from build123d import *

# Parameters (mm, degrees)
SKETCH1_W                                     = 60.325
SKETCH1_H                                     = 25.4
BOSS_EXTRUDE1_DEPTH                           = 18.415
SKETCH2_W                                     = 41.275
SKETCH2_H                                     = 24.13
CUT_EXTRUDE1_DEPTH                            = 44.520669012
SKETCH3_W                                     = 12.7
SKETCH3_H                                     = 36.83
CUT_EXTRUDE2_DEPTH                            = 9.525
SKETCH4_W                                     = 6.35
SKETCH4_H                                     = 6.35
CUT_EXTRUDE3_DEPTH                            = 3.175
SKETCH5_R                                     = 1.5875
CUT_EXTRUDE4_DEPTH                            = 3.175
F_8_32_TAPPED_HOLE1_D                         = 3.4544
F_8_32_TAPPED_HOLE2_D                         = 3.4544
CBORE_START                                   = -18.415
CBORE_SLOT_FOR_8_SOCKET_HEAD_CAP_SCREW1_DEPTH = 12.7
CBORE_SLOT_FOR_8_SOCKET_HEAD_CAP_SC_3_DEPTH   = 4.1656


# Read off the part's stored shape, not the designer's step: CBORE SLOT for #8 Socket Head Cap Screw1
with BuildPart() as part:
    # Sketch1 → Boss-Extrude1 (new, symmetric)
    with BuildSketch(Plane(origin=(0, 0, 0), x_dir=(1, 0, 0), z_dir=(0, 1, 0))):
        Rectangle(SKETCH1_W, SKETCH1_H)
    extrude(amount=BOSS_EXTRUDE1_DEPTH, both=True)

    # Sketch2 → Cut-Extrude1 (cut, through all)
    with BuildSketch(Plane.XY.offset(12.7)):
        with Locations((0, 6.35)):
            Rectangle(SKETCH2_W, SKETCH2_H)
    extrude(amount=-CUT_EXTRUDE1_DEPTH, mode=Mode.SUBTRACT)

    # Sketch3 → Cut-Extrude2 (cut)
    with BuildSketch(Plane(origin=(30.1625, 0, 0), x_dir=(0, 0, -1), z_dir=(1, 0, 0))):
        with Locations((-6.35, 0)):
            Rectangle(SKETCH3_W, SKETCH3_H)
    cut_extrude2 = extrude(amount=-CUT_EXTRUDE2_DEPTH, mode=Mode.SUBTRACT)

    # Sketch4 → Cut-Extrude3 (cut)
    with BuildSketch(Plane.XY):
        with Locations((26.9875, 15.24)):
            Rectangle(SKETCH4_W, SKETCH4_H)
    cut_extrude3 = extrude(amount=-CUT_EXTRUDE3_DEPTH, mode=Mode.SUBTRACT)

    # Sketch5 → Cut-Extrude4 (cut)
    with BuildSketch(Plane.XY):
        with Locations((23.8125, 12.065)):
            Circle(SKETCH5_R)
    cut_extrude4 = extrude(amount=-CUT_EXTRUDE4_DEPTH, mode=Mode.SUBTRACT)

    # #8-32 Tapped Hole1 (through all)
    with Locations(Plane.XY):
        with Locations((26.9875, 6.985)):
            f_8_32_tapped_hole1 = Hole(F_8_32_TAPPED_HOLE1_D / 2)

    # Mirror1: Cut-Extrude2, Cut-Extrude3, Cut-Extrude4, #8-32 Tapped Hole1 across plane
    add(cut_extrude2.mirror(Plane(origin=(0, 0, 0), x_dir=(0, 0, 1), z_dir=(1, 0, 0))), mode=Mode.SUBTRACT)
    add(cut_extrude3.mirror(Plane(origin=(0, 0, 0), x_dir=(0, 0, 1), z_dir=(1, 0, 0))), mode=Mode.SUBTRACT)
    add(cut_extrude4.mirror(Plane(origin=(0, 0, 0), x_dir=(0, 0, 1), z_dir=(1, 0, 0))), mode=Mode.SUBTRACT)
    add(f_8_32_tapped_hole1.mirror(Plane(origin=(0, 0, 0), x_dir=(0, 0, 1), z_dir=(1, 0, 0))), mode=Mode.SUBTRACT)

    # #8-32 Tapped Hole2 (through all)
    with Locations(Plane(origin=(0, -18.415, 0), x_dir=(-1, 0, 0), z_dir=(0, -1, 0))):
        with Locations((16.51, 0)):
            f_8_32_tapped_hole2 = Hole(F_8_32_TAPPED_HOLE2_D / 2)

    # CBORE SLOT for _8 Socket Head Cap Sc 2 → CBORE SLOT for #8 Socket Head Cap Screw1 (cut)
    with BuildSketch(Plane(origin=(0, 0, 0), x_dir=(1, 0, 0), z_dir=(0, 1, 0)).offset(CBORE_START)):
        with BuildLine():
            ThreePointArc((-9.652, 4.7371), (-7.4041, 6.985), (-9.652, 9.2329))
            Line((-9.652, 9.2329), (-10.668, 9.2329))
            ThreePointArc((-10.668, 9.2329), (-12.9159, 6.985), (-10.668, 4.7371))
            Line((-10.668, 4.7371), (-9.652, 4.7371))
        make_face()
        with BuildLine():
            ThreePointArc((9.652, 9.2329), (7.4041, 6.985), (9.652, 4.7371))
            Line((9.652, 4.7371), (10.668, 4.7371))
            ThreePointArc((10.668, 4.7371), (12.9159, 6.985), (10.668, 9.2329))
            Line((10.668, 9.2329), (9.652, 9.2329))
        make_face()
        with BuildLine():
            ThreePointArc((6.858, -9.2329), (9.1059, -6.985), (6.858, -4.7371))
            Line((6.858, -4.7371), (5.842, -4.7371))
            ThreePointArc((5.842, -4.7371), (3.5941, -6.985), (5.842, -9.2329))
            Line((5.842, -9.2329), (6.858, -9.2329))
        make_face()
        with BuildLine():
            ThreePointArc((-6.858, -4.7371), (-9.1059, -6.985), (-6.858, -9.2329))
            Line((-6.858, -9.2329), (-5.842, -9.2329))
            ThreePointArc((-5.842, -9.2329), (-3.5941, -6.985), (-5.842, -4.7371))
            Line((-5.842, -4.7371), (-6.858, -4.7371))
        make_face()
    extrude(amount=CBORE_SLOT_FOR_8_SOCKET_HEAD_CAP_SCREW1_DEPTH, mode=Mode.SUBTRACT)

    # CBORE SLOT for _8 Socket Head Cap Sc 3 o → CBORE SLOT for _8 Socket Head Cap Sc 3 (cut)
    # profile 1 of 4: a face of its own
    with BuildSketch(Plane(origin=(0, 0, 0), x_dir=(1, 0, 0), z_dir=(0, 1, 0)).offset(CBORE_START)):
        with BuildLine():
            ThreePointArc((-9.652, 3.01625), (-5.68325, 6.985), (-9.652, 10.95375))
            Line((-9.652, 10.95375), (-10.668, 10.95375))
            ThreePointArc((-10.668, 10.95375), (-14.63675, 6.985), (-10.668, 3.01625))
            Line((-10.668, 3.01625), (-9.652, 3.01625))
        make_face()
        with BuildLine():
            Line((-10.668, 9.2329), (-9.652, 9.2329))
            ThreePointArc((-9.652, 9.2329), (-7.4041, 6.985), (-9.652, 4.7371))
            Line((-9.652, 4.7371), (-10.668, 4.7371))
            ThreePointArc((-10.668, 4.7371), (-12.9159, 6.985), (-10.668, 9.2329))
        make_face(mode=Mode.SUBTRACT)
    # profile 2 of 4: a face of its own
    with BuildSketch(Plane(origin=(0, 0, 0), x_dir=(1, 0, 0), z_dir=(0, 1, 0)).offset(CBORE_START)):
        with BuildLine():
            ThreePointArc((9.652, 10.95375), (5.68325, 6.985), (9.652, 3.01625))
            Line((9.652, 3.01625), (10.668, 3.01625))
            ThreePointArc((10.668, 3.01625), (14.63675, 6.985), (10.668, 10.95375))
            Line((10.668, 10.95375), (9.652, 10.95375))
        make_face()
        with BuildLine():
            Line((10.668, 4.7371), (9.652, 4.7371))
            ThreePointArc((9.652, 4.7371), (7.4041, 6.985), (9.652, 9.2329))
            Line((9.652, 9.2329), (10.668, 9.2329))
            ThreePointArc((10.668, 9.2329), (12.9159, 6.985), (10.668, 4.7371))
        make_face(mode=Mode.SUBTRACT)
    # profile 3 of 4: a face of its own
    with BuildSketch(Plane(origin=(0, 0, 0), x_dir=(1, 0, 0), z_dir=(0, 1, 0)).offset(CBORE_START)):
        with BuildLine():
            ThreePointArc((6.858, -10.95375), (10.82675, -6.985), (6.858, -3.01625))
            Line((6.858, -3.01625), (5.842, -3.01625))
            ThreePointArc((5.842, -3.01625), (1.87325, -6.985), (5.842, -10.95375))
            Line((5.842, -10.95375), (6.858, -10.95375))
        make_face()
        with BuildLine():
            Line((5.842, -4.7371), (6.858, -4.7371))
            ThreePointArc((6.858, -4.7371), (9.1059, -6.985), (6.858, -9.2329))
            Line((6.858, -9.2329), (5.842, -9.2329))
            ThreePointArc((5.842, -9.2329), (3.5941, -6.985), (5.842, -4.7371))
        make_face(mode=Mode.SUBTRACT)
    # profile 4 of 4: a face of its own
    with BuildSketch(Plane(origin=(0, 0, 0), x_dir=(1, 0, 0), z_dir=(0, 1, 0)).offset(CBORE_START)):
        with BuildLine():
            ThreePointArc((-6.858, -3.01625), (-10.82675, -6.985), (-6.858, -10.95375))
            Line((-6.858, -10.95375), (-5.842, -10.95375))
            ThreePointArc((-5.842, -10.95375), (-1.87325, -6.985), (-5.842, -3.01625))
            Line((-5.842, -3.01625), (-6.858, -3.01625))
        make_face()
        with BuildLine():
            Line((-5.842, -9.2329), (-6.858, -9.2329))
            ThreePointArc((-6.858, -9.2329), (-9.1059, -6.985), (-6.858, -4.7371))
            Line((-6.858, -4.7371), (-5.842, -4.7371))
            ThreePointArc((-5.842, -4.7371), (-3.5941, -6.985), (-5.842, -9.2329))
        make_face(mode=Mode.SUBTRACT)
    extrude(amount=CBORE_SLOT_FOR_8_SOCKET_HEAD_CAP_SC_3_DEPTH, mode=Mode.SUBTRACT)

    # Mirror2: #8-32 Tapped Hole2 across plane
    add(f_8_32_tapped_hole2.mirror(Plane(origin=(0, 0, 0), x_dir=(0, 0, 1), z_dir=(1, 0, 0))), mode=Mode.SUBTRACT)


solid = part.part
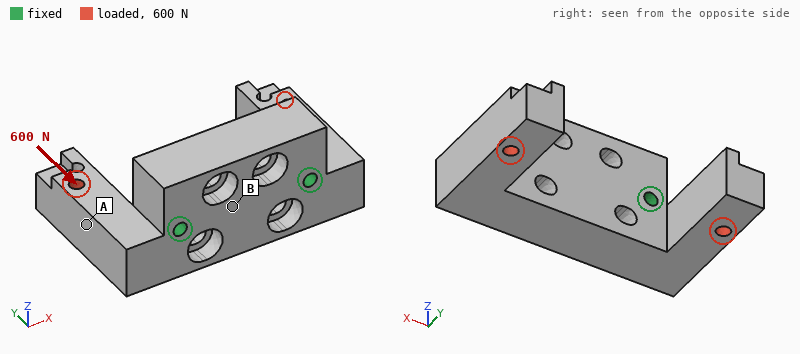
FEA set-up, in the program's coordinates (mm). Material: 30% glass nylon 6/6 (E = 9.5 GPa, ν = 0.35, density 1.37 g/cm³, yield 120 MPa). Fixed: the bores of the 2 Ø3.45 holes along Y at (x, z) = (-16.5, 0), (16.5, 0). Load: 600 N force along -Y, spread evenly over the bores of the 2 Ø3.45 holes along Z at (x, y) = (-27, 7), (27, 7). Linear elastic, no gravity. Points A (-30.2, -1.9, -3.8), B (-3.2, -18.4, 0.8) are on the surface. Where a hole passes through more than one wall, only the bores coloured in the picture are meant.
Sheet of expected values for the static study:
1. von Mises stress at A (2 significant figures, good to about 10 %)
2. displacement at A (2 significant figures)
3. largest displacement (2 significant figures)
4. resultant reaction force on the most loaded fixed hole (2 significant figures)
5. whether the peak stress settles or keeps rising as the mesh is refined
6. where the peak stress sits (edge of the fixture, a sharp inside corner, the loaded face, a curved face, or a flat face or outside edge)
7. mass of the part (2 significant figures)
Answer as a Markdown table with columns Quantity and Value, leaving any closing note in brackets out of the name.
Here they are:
| Quantity | Value |
|---|---|
| von Mises stress at A | 5.2 MPa |
| displacement at A | 31 µm |
| largest displacement | 75 µm |
| resultant reaction force on the most loaded fixed hole | 300 N |
| whether the peak stress settles or keeps rising as the mesh is refined | keeps rising |
| where the peak stress sits | edge of the fixture |
| mass of the part | 27 g |
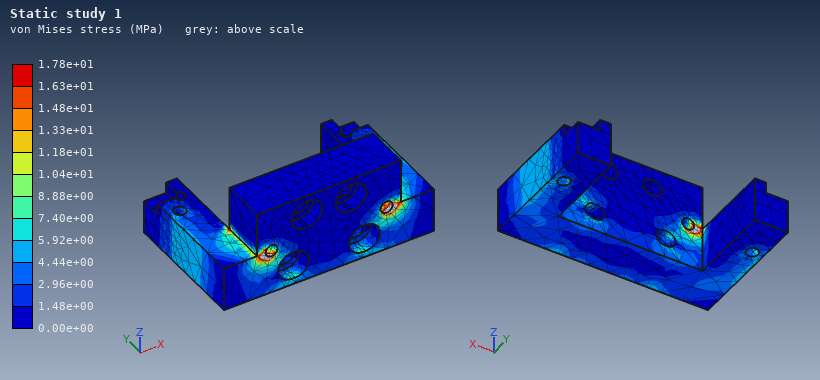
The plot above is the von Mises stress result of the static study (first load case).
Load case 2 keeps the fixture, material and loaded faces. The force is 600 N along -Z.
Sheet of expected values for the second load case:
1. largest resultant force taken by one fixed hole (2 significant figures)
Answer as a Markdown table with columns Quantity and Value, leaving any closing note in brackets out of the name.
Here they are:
| Quantity | Value |
|---|---|
| largest resultant force taken by one fixed hole | 340 N |
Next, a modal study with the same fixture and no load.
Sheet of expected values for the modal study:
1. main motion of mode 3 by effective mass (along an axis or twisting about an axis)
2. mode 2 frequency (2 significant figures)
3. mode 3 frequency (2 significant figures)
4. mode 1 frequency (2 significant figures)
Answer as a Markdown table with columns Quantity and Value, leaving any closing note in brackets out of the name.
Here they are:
| Quantity | Value |
|---|---|
| main motion of mode 3 by effective mass | along Z |
| mode 2 frequency | 3800 Hz |
| mode 3 frequency | 4100 Hz |
| mode 1 frequency | 3700 Hz |
